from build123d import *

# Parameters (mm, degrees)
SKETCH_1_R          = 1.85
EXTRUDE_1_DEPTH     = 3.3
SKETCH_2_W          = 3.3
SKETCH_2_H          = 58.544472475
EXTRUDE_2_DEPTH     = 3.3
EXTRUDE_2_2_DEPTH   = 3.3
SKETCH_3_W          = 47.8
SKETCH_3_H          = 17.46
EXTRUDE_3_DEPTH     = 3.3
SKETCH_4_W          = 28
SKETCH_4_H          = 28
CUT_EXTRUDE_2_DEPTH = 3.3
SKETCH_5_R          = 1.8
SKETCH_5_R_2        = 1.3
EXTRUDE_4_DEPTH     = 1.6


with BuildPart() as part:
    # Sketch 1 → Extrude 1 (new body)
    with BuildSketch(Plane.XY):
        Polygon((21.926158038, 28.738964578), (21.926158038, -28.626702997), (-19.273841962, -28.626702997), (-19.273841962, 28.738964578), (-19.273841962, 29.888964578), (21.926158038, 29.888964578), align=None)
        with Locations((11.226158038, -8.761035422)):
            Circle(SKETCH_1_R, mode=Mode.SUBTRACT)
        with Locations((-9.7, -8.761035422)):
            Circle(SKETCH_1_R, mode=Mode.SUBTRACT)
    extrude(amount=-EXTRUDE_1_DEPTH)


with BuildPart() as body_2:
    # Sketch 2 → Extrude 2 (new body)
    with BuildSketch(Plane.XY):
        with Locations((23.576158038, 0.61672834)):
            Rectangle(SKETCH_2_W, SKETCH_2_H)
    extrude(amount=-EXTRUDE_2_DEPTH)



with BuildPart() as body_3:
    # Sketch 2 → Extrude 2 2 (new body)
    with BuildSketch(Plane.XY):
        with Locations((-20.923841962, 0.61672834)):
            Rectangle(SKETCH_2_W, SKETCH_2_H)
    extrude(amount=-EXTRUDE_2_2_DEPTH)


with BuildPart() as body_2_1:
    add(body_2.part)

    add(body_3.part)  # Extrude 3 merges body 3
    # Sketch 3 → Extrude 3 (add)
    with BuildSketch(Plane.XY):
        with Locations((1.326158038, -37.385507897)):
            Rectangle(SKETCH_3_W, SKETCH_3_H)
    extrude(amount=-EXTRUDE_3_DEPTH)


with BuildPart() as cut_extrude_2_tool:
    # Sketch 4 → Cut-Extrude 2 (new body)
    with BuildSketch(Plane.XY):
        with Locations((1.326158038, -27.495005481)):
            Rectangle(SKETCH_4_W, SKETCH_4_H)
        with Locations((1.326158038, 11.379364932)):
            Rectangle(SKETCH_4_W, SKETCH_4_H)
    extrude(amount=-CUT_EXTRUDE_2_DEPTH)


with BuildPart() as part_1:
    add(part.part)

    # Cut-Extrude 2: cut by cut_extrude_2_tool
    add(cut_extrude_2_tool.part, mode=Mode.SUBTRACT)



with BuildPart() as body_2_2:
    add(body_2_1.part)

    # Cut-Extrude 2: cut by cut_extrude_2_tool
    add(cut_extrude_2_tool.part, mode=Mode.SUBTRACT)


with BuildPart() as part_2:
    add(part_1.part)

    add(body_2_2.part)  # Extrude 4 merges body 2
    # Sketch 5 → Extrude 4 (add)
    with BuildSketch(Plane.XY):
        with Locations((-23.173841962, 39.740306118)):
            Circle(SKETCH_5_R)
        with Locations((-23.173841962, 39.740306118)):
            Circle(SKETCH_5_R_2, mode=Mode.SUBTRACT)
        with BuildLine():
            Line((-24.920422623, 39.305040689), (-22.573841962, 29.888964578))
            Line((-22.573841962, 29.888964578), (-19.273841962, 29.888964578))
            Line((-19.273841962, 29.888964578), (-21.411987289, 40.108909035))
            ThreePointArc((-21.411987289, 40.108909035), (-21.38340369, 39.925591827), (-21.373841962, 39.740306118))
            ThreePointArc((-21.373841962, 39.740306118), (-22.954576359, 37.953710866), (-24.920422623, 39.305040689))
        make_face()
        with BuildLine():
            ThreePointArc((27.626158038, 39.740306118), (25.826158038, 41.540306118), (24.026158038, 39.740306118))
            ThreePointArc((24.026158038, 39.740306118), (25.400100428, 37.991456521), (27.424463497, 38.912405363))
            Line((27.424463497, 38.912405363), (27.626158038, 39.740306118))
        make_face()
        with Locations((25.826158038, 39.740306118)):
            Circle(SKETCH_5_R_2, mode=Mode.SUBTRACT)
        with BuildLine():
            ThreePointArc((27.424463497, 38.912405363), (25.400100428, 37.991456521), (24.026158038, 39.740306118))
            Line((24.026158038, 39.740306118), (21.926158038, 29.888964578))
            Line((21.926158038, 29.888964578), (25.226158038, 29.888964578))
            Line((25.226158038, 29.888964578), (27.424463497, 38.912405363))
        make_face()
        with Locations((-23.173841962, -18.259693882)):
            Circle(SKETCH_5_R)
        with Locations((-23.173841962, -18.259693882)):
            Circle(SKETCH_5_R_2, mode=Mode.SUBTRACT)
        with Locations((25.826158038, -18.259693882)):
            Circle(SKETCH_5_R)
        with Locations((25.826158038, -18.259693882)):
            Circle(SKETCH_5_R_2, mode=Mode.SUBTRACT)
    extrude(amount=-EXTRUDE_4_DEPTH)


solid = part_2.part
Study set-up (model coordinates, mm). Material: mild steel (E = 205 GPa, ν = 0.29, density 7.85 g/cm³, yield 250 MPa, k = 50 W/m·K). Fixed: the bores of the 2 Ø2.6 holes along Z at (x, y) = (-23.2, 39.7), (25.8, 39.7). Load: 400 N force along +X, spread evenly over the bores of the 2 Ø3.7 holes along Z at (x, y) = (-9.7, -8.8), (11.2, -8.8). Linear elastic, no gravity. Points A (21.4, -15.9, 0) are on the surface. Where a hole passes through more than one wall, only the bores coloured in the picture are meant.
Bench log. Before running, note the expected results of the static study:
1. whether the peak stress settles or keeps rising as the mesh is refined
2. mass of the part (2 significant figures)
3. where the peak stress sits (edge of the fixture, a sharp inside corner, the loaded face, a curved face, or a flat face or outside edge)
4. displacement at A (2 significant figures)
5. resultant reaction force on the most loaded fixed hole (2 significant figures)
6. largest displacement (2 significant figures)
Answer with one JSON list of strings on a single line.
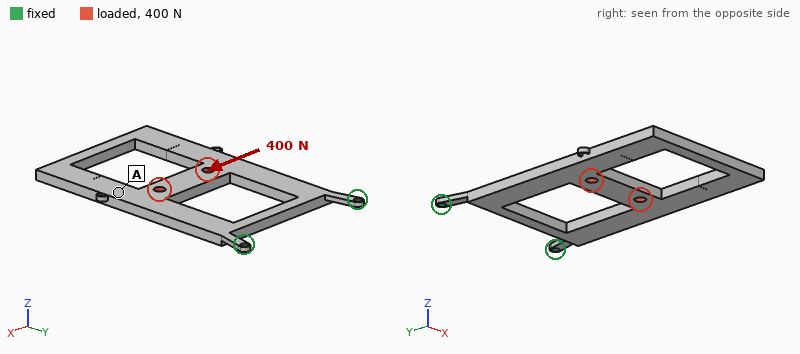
["keeps rising", "54 g", "edge of the fixture", "61 µm", "410 N", "64 µm"]
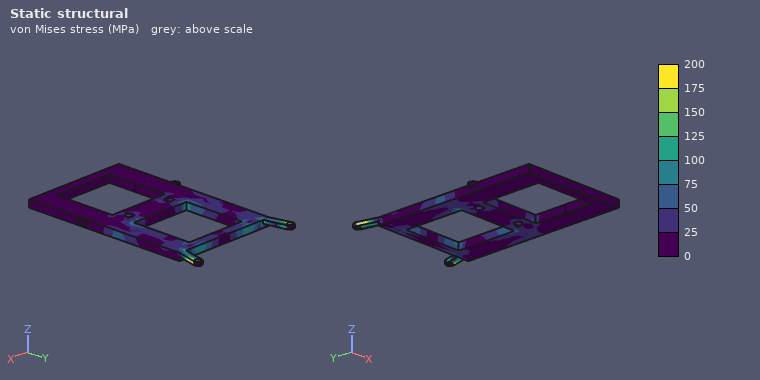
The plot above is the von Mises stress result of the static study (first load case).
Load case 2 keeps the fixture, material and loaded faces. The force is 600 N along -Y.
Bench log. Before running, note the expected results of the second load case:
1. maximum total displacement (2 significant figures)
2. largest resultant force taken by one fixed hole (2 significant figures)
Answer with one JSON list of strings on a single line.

["0.82 mm", "310 N"]
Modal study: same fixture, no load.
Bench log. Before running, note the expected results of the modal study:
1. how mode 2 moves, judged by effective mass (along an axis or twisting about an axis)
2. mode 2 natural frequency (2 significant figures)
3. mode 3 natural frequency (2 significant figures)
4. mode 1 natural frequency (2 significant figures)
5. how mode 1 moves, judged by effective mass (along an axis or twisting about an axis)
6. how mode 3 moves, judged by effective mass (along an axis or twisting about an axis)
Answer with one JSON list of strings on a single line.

["twisting about Y", "850 Hz", "1400 Hz", "98 Hz", "along Z", "along Z"]
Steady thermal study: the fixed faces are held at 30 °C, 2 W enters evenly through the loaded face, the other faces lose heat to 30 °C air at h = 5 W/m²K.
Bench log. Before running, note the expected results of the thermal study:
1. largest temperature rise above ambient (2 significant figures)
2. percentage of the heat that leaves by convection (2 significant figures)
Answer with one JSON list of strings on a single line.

["39 K", "45 %"]
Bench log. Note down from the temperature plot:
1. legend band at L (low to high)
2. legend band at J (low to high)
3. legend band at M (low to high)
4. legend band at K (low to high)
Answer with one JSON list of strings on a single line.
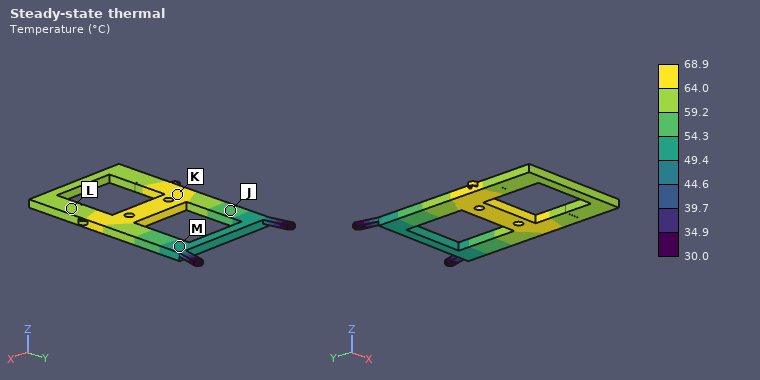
["59.2 to 64.0 °C", "54.3 to 59.2 °C", "49.4 to 54.3 °C", "64.0 to 68.9 °C"]
